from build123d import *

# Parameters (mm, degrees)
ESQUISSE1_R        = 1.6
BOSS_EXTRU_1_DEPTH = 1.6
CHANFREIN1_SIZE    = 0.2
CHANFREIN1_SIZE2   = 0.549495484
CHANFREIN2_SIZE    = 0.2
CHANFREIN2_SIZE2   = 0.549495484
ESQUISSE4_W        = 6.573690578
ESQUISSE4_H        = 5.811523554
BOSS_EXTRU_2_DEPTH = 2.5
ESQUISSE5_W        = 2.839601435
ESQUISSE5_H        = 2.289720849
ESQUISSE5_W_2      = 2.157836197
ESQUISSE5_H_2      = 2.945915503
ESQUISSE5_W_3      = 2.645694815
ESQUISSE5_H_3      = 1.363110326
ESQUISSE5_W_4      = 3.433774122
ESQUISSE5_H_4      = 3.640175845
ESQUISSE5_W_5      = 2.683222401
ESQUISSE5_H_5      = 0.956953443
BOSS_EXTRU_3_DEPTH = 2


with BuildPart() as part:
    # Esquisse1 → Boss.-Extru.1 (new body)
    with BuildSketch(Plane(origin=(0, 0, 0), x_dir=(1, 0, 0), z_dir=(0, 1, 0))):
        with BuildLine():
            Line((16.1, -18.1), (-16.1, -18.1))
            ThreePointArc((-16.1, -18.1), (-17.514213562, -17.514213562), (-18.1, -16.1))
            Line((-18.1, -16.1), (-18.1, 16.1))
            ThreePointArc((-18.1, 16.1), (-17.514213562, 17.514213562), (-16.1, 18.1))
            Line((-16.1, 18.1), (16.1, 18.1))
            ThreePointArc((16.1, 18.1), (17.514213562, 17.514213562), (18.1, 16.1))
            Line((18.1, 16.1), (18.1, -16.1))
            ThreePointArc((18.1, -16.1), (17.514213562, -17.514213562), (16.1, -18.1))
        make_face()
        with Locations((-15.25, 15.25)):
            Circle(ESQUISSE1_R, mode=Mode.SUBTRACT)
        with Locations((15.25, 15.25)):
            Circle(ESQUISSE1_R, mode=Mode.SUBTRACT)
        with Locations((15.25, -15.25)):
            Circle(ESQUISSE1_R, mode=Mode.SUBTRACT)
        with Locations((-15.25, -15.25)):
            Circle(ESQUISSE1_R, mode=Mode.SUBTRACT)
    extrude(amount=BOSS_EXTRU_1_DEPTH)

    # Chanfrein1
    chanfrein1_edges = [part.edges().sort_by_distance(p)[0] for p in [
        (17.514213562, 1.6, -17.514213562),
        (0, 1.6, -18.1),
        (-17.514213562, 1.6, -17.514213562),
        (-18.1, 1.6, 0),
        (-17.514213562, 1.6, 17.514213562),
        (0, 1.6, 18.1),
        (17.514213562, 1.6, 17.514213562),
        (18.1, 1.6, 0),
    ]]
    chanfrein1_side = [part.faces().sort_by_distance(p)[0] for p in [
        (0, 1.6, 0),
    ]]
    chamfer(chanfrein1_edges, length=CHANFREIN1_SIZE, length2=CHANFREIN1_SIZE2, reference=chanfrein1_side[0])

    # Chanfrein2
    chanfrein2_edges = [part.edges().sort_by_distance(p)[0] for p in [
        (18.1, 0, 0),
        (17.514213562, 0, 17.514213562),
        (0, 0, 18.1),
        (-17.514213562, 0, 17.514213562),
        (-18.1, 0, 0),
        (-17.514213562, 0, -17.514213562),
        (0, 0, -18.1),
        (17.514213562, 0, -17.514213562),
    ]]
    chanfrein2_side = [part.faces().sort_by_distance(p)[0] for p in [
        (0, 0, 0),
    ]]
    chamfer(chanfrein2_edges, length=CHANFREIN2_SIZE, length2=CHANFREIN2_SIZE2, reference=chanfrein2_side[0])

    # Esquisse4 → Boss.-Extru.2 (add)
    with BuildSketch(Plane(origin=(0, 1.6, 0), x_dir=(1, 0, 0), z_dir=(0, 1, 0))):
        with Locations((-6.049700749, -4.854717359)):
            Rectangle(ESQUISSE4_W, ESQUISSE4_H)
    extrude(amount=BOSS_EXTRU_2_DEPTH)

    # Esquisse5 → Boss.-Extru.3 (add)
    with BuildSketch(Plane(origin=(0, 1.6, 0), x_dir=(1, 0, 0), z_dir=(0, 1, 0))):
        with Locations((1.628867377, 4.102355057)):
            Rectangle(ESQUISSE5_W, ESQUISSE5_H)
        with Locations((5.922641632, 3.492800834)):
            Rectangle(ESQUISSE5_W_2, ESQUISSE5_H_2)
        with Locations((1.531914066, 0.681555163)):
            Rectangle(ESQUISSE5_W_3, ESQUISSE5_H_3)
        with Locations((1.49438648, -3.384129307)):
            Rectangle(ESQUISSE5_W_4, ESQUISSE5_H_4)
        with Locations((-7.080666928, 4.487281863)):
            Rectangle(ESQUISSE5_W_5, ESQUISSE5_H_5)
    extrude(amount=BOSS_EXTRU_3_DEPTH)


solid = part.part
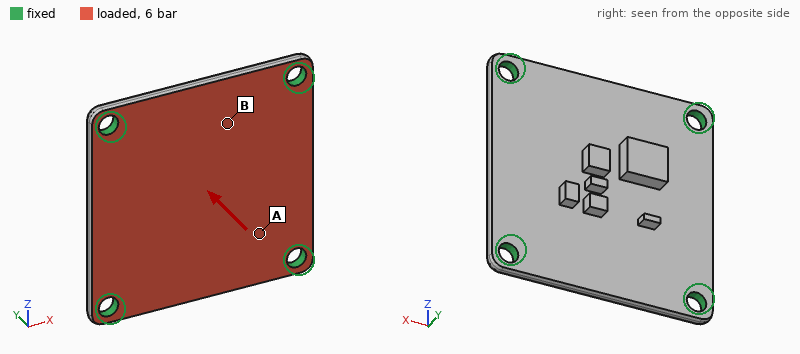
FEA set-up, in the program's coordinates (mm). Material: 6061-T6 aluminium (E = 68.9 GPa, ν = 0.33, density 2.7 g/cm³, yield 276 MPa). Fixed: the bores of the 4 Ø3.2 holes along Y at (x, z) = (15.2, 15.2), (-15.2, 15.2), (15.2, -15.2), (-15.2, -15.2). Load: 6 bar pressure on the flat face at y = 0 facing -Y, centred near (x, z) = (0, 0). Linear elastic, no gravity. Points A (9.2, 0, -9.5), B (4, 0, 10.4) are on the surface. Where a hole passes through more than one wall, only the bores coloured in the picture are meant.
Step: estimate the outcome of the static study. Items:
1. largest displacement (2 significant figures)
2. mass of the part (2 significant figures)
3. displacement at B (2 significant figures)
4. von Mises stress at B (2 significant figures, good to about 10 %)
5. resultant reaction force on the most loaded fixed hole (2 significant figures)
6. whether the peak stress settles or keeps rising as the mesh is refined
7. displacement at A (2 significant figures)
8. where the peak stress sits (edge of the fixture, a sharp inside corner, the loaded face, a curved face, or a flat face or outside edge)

0.12 mm
5.9 g
0.076 mm
49 MPa
190 N
keeps rising
0.055 mm
edge of the fixture
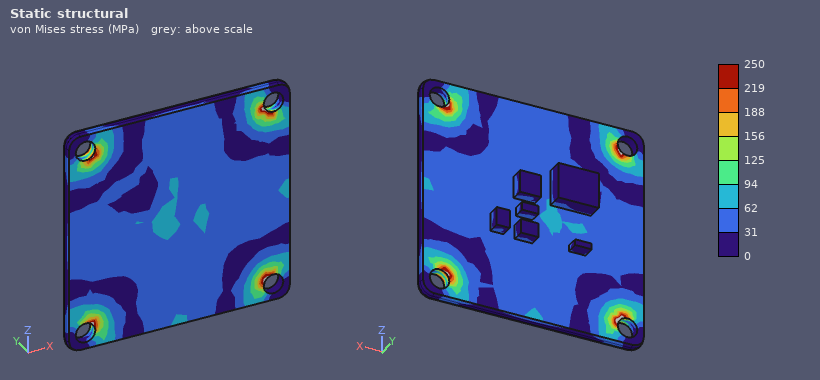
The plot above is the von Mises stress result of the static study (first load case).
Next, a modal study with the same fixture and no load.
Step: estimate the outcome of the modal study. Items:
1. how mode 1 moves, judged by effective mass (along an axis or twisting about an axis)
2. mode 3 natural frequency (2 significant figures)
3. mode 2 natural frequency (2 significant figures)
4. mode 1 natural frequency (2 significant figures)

along Y
11 kHz
11 kHz
6200 Hz
